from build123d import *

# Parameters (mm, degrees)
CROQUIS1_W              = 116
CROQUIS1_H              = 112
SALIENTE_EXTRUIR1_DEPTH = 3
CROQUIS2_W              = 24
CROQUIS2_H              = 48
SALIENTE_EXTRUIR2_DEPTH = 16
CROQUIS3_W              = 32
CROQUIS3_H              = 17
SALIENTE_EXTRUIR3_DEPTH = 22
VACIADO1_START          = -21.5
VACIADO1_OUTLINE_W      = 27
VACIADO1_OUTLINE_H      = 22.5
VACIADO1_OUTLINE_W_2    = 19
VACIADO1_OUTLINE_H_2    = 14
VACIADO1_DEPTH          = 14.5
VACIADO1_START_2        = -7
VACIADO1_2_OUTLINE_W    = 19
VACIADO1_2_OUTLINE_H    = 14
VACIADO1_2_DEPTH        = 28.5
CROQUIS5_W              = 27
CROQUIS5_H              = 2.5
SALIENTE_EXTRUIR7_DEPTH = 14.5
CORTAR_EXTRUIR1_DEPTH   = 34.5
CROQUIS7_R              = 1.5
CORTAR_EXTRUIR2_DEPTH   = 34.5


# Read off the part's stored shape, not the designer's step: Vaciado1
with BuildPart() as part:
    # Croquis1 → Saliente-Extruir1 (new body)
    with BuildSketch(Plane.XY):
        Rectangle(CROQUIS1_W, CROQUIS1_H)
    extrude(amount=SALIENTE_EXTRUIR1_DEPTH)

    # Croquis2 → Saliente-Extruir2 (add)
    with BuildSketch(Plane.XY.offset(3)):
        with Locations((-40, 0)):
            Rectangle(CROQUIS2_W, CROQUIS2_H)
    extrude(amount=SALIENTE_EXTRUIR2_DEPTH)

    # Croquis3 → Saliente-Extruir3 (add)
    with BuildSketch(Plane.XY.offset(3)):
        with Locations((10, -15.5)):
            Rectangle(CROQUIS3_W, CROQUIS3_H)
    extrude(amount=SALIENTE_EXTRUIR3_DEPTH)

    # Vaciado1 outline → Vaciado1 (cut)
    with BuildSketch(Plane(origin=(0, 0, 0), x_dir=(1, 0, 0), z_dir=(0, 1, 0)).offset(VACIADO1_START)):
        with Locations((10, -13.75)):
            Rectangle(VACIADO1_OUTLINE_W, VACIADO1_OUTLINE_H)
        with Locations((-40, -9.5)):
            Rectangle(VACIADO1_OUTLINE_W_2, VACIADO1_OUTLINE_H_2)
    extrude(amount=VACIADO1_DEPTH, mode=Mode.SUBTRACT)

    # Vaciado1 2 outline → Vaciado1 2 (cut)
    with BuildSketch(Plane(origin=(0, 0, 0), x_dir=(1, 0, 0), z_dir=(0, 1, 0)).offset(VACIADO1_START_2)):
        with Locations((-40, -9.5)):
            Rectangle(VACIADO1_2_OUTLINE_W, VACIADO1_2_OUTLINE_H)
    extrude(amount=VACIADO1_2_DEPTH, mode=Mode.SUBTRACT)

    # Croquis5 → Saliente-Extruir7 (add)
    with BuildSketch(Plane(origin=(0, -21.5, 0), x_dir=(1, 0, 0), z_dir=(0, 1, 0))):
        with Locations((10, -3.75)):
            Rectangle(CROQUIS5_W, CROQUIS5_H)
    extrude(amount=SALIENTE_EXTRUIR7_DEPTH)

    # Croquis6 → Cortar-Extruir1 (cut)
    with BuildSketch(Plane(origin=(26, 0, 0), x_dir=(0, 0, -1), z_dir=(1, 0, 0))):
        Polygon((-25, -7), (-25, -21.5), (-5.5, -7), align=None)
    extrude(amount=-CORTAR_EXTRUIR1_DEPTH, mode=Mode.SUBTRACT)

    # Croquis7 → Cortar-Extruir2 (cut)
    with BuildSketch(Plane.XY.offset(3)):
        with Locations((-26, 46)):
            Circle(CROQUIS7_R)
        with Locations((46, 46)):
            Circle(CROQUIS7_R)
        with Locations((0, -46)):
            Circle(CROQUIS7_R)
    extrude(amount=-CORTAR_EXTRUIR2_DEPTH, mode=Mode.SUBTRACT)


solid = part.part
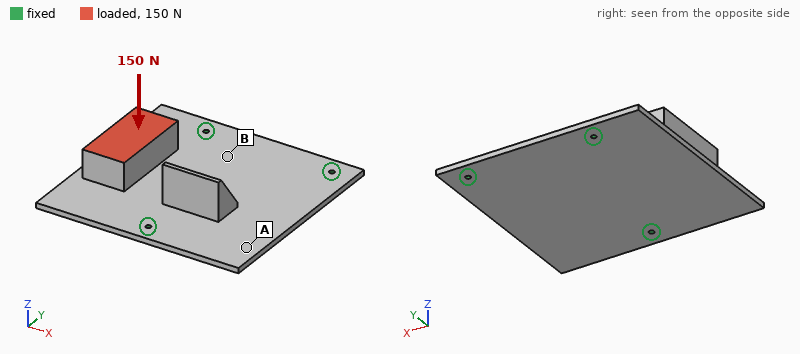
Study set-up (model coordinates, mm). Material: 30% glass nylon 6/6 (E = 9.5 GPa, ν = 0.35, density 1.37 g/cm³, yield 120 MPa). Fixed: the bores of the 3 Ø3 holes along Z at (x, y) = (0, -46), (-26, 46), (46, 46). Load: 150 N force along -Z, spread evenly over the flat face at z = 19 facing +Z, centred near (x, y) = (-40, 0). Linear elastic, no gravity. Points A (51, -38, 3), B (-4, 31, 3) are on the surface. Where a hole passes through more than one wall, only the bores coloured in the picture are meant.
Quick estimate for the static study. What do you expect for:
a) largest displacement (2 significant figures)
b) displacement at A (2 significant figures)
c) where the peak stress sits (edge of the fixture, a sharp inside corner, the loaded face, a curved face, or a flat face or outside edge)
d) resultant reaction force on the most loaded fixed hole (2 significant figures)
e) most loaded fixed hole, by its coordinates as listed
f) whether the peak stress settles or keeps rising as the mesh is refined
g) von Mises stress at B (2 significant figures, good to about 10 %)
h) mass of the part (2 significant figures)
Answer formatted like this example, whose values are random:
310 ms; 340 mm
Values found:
1.6 mm; 0.43 mm; edge of the fixture; 110 N; (-26, 46); keeps rising; 6.2 MPa; 68 g
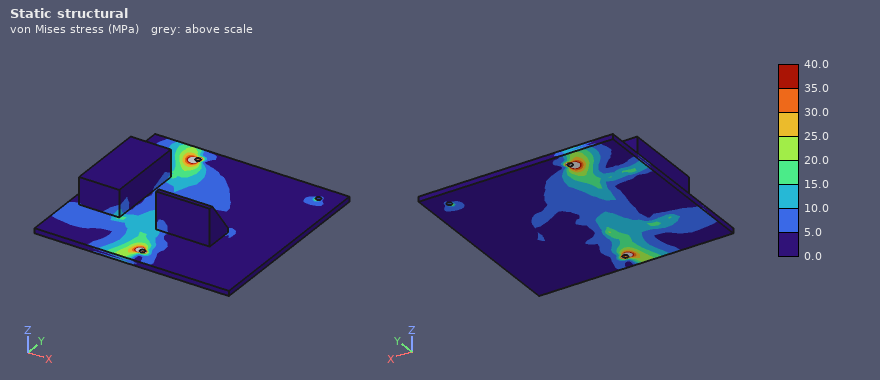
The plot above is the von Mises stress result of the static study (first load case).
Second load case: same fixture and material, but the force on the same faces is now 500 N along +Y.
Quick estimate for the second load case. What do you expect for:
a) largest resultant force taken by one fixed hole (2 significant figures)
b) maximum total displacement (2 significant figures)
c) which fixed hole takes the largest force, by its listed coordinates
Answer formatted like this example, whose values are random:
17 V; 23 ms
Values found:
310 N; 1.6 mm; (-26, 46)
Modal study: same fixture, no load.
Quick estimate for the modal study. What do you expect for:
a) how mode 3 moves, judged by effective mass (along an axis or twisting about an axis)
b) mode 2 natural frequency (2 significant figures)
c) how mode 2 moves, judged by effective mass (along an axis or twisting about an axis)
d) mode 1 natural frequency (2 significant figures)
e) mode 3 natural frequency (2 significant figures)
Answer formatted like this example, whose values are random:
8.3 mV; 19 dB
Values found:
along Z; 500 Hz; along Z; 360 Hz; 840 Hz
